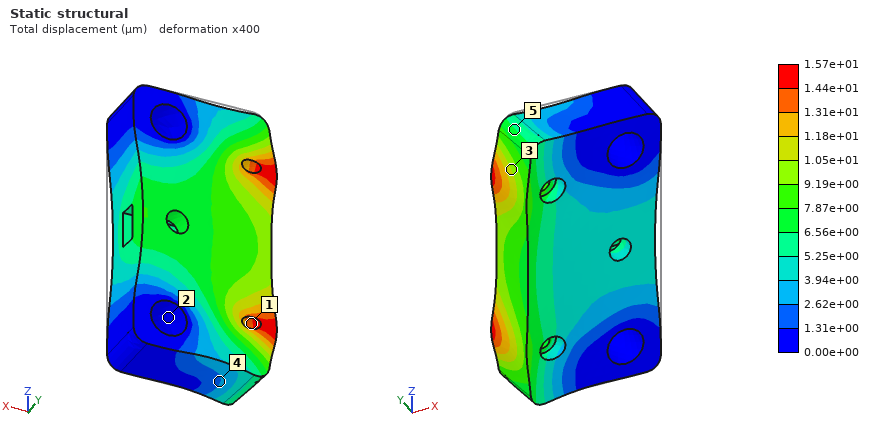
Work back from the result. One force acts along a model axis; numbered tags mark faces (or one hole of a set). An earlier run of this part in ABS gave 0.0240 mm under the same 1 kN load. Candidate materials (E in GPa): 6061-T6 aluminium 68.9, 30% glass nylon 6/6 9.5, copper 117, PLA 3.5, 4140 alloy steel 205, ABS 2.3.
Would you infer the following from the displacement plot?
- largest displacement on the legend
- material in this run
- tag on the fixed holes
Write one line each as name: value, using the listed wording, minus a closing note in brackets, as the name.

largest displacement on the legend: 1.57e+01 µm
material in this run: PLA
tag on the fixed holes: 2
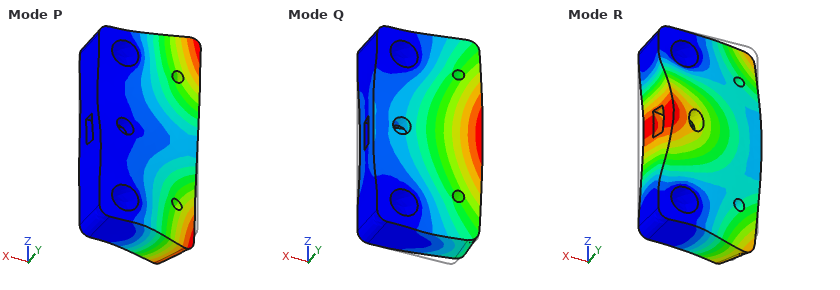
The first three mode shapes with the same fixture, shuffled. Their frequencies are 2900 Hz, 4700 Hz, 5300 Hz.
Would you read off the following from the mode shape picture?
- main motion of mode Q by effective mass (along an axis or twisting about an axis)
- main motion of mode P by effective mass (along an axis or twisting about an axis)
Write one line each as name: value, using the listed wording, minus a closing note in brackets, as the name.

main motion of mode Q by effective mass: along Y
main motion of mode P by effective mass: twisting about X
